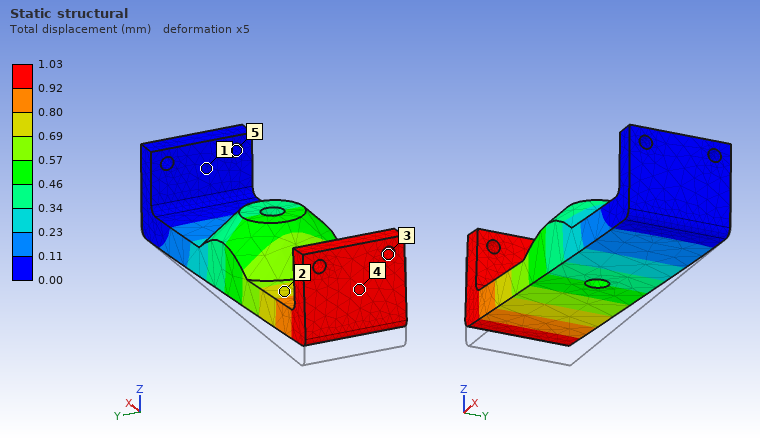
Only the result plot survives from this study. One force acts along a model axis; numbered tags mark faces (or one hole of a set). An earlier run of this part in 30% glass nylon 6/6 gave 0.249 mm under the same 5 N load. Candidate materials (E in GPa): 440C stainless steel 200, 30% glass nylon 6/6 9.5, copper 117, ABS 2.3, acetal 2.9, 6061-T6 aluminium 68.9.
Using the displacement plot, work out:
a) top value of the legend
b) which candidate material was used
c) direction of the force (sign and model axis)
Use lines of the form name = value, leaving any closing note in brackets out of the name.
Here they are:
top value of the legend = 1.03 mm
which candidate material was used = ABS
direction of the force = +Z
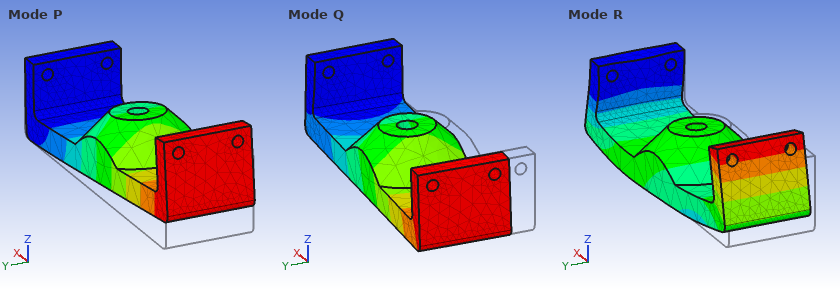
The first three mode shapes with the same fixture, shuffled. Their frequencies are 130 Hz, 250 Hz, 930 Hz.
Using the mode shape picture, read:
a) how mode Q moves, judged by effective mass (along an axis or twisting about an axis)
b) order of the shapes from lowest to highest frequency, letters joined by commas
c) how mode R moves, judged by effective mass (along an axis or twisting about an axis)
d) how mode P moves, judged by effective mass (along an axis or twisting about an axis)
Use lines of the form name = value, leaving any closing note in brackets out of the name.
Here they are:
how mode Q moves, judged by effective mass = along Y
order of the shapes from lowest to highest frequency, letters joined by commas = P, Q, R
how mode R moves, judged by effective mass = along X
how mode P moves, judged by effective mass = along Z
